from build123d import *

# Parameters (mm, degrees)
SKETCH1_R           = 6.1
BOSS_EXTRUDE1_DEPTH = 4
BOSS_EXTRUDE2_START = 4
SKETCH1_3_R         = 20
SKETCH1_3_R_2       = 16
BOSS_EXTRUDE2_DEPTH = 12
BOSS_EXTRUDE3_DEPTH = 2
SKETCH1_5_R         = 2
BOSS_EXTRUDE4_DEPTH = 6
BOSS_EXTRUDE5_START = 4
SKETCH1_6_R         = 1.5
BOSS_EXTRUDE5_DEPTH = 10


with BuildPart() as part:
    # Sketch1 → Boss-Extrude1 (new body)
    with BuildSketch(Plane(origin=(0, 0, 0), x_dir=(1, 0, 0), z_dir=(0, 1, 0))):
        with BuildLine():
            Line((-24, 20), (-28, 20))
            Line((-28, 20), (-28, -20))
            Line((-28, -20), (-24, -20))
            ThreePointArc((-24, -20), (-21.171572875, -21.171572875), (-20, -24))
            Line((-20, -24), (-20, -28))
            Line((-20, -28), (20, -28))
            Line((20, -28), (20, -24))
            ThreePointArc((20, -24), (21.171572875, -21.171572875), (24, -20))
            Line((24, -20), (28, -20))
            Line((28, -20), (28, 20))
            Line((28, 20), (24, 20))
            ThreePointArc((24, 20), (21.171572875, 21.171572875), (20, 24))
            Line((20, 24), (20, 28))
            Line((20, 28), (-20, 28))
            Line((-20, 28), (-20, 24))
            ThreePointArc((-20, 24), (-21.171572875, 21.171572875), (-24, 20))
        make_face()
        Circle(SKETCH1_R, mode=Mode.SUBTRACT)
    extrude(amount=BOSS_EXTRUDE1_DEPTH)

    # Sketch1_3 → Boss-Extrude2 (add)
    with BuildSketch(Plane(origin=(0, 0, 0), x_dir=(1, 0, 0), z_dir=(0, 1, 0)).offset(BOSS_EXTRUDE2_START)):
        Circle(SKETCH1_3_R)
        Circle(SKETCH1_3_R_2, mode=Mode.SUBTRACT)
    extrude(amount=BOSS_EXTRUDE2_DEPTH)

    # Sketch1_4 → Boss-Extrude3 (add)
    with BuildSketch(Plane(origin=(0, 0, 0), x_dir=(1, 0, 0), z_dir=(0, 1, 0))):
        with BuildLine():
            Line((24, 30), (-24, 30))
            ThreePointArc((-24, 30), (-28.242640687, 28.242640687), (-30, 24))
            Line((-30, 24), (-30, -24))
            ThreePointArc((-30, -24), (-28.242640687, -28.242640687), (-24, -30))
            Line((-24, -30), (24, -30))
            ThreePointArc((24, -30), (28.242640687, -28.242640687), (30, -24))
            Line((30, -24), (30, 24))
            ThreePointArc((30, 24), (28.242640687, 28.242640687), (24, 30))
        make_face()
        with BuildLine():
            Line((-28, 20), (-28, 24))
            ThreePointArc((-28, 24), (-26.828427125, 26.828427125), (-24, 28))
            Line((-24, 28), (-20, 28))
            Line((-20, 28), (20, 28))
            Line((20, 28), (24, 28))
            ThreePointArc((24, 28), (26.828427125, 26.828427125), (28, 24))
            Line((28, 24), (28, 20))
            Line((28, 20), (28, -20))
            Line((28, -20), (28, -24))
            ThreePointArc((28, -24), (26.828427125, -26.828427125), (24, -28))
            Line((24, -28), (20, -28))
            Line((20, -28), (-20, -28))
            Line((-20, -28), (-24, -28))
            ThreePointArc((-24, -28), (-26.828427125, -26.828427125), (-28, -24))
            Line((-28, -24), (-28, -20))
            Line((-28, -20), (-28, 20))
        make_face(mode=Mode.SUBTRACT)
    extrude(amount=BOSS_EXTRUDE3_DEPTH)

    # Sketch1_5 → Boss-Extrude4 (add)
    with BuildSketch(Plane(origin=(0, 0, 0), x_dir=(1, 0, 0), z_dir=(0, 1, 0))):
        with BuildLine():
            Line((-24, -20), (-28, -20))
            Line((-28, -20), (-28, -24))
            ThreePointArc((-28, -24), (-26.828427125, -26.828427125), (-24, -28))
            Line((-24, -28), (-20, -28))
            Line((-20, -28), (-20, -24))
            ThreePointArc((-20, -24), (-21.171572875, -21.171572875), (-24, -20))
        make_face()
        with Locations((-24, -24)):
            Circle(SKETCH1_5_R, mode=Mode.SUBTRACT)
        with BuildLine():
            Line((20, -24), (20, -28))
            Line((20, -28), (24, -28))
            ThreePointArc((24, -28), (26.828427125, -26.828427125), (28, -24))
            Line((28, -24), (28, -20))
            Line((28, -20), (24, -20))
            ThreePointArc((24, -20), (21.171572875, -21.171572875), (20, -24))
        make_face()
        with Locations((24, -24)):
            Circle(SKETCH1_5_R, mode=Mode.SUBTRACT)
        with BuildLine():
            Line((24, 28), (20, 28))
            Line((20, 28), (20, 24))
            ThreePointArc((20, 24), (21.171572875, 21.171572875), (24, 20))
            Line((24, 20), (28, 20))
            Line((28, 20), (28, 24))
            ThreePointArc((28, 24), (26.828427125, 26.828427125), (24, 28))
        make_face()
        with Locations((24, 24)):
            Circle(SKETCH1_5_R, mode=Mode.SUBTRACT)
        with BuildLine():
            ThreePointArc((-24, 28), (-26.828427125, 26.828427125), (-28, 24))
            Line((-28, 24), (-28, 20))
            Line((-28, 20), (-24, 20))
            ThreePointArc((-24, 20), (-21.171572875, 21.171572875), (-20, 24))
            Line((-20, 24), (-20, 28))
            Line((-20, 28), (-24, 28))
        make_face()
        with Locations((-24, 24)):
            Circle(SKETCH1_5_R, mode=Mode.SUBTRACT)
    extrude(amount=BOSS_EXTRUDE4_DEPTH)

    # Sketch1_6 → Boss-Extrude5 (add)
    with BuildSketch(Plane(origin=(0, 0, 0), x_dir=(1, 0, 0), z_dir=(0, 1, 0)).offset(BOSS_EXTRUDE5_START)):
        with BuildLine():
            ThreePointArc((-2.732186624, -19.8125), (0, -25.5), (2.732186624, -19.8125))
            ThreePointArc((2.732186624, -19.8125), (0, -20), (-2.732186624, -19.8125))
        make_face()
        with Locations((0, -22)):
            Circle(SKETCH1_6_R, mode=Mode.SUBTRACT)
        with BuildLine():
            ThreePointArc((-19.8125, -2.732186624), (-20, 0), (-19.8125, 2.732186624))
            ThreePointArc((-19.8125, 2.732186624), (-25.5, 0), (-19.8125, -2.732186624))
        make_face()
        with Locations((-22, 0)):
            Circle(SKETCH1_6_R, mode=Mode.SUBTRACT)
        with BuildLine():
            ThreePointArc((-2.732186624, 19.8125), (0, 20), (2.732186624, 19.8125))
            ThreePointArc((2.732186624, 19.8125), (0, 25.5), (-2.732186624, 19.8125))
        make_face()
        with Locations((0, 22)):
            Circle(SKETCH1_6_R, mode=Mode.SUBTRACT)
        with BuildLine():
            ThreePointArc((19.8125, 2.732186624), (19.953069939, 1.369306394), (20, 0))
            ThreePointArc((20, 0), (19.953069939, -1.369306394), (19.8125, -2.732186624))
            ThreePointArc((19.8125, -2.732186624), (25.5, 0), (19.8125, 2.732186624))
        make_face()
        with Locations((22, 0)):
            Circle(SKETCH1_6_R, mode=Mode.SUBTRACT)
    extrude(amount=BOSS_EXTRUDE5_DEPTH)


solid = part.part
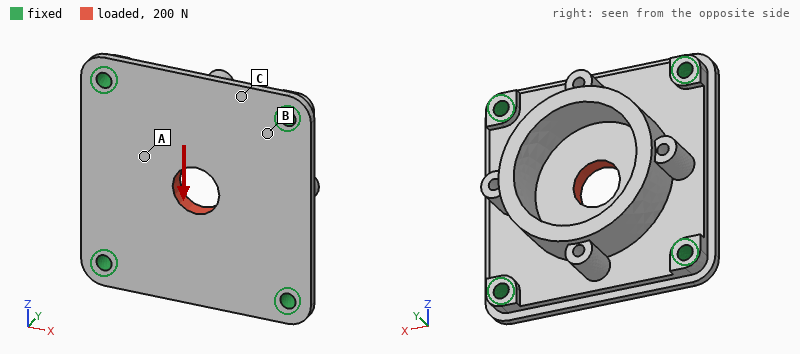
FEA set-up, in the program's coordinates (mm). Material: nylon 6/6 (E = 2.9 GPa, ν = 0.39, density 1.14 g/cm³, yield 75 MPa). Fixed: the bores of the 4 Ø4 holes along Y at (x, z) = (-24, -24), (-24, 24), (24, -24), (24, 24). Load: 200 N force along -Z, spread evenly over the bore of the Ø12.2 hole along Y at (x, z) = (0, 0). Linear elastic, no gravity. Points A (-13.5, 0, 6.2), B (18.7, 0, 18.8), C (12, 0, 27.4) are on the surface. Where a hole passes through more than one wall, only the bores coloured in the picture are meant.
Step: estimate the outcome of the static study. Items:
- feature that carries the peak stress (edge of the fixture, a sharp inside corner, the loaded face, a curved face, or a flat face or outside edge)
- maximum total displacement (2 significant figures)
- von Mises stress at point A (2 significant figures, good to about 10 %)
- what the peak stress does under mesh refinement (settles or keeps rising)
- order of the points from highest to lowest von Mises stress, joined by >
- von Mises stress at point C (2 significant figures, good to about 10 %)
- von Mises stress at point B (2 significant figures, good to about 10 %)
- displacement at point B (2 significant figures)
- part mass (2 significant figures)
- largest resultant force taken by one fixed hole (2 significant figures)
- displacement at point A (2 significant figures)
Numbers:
edge of the fixture
13 µm
0.73 MPa
keeps rising
B > A > C
0.32 MPa
1.1 MPa
3.7 µm
22 g
56 N
6.8 µm
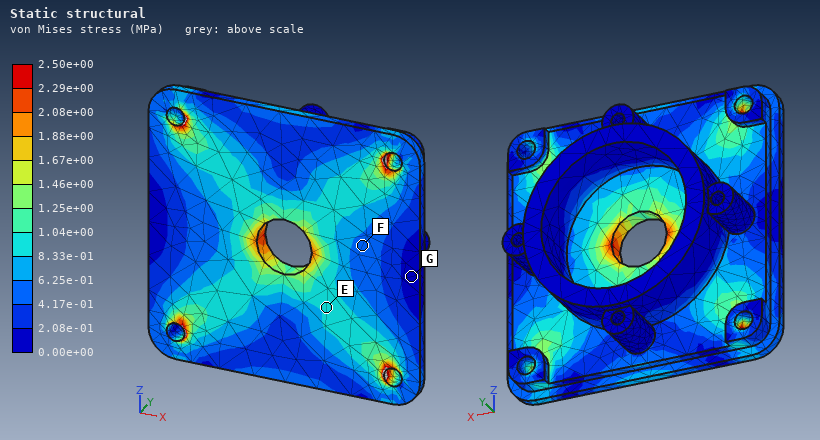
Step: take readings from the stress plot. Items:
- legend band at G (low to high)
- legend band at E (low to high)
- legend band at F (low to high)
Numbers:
0.00e+00 to 2.08e-01 MPa
8.33e-01 to 1.04e+00 MPa
4.17e-01 to 6.25e-01 MPa
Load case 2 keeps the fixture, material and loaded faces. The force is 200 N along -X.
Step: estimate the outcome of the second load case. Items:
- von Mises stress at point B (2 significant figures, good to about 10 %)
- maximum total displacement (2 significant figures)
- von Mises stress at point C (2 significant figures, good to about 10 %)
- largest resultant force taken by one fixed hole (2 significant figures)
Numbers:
1.1 MPa
13 µm
0.32 MPa
56 N
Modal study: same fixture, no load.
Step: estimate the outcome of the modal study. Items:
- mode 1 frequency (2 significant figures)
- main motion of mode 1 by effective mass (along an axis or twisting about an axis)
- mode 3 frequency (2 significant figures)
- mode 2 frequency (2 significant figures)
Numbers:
2200 Hz
along Y
2900 Hz
2900 Hz
